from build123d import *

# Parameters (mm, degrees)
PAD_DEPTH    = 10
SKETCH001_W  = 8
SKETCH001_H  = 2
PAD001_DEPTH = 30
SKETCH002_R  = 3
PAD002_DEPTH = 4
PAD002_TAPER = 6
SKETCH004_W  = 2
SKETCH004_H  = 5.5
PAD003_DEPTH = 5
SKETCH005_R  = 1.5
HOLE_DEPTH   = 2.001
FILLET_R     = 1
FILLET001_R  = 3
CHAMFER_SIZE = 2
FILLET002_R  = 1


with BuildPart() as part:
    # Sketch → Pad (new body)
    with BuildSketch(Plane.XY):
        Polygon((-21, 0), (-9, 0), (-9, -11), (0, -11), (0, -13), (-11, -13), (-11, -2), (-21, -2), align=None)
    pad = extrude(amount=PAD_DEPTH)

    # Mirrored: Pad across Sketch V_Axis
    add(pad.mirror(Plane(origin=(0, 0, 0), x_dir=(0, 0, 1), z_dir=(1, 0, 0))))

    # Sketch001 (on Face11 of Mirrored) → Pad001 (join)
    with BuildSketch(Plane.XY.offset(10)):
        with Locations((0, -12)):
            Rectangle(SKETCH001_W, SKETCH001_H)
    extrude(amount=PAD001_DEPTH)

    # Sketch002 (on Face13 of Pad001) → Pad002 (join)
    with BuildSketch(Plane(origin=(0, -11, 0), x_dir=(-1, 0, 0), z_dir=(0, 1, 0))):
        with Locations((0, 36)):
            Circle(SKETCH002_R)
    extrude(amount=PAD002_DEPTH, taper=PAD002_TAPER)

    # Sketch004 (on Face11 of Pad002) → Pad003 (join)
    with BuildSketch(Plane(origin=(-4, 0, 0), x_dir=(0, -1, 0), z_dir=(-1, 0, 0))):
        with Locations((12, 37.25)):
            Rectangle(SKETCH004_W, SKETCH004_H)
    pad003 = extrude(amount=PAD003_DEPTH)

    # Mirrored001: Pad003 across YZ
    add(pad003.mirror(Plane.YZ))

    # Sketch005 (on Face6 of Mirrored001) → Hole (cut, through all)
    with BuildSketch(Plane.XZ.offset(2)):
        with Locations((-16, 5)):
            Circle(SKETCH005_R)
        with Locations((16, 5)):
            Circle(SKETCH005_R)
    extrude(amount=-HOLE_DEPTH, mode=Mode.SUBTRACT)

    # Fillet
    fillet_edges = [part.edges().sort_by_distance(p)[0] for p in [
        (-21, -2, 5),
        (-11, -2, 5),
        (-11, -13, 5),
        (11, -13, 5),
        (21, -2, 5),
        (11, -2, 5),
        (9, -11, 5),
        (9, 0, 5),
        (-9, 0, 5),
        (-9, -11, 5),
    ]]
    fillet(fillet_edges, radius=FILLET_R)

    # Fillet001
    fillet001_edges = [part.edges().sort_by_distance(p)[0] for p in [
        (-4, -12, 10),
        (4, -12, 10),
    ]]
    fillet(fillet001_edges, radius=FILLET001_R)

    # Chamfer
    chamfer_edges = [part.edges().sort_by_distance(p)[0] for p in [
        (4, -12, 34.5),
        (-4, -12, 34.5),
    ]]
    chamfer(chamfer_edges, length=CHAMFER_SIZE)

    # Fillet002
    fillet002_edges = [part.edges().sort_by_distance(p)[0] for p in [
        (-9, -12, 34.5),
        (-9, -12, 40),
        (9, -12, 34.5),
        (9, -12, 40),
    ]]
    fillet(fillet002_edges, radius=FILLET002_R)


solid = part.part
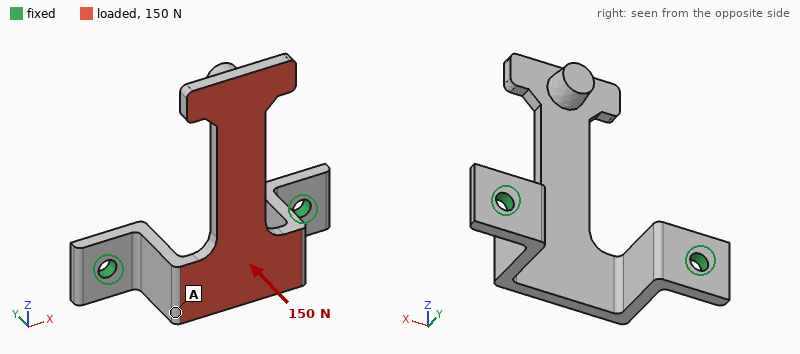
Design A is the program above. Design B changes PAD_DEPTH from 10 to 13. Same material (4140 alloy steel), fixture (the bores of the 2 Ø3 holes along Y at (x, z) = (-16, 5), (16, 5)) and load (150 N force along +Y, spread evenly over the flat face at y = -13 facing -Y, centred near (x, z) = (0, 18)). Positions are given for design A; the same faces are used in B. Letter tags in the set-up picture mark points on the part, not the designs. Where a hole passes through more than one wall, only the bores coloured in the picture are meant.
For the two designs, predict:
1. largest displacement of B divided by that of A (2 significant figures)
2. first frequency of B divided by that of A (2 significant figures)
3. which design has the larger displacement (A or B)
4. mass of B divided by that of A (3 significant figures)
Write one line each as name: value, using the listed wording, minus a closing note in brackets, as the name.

largest displacement of B divided by that of A: 0.66
first frequency of B divided by that of A: 1.2
which design has the larger displacement: A
mass of B divided by that of A: 1.17
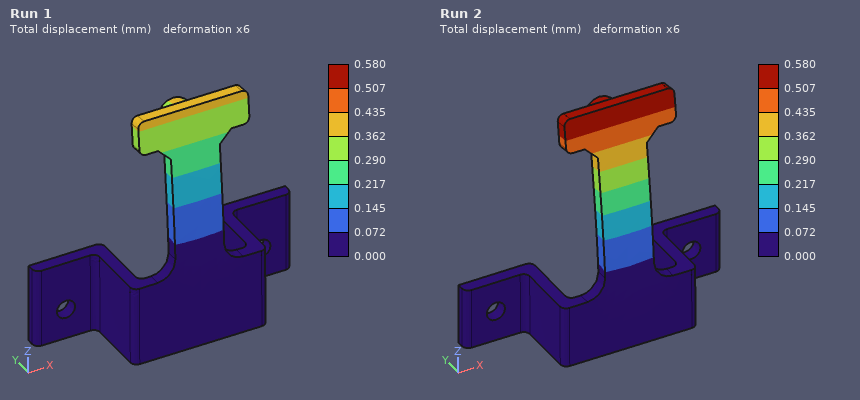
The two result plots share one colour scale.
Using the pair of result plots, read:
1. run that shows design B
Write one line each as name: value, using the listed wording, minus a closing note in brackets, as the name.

run that shows design B: Run 1
